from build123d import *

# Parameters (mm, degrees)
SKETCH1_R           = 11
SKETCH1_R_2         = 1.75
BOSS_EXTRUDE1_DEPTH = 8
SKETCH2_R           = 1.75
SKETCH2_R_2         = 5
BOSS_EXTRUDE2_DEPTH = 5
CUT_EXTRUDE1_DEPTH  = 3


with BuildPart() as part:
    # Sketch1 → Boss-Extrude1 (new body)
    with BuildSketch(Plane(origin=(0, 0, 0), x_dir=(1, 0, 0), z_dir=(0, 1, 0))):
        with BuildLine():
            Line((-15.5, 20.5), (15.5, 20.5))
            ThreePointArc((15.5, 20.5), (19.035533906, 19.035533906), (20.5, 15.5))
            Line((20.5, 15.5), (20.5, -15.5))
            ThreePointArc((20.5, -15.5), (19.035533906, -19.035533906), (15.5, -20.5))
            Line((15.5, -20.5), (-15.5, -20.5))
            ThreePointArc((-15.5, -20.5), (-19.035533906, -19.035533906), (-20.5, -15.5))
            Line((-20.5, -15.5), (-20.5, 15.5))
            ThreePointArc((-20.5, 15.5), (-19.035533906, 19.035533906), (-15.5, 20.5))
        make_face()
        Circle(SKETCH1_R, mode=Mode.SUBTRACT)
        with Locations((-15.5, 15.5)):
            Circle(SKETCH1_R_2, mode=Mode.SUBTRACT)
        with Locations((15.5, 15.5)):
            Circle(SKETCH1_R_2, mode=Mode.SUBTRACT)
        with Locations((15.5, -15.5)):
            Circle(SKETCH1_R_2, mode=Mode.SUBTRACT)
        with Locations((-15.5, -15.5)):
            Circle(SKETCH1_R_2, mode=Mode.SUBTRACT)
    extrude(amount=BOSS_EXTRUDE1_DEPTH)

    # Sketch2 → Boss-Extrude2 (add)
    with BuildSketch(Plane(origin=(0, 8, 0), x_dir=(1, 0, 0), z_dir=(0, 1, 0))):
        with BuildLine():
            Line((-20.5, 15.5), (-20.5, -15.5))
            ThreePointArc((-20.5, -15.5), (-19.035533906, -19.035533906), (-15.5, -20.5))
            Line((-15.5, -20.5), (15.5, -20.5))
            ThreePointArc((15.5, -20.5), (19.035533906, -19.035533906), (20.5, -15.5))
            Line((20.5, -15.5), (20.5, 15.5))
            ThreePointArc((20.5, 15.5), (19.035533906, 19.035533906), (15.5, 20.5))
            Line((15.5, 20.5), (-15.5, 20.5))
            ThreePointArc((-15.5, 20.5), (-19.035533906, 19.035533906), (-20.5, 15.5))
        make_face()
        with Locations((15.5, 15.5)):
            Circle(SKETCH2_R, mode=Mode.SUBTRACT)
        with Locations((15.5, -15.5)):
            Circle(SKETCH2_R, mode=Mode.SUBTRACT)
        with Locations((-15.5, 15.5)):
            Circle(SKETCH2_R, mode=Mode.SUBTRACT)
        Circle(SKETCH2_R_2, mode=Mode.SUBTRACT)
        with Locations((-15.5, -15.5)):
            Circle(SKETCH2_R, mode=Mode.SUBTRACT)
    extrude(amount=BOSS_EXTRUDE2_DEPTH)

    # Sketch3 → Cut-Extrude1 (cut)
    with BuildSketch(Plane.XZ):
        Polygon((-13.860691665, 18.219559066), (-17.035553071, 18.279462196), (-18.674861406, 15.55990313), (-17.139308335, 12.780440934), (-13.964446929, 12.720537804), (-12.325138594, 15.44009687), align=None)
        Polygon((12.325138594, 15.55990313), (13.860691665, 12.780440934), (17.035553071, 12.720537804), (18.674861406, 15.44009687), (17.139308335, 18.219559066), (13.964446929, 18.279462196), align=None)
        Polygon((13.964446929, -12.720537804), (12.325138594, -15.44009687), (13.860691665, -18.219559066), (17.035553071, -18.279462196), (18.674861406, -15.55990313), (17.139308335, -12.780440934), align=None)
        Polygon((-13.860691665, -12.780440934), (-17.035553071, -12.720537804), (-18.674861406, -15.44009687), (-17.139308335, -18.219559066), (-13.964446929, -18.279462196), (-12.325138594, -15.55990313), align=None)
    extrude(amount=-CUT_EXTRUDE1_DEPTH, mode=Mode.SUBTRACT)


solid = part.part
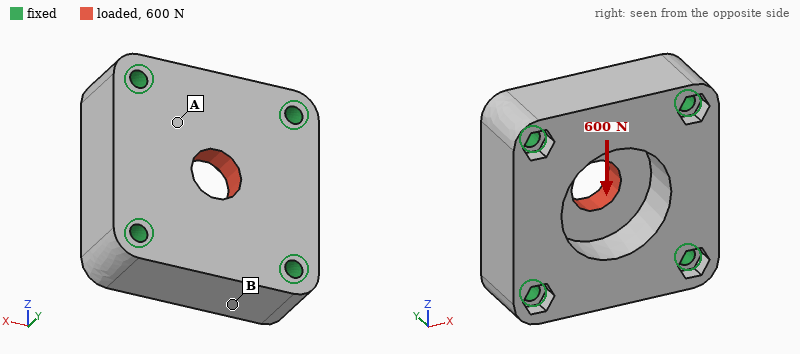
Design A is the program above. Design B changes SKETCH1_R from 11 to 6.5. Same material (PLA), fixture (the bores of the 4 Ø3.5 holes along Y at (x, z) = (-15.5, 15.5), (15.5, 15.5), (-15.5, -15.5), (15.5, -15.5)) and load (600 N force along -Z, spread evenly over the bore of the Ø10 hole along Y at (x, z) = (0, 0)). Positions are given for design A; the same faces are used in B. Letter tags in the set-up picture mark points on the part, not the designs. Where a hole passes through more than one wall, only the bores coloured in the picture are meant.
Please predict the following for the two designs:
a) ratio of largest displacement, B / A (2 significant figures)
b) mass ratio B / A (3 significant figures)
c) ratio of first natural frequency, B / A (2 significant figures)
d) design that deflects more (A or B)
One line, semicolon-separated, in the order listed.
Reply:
0.91; 1.11; 0.94; A
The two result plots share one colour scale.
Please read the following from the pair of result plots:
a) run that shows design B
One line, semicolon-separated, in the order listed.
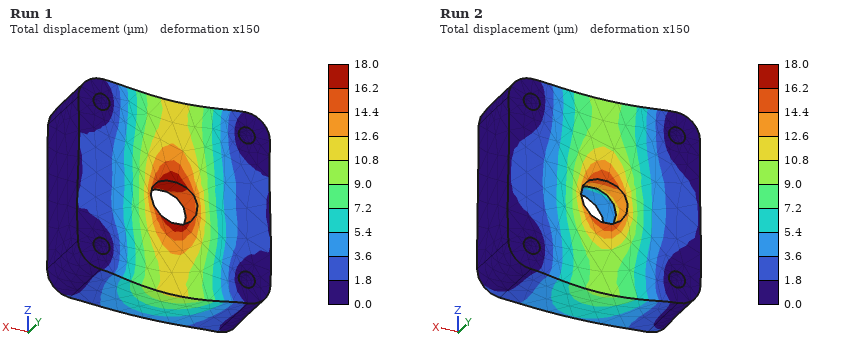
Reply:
Run 2
